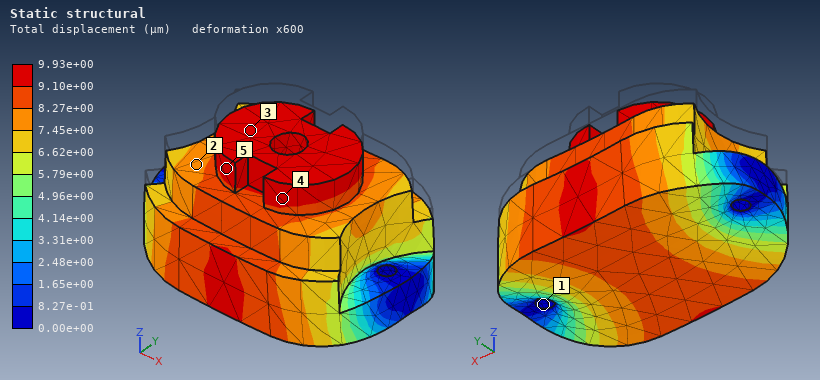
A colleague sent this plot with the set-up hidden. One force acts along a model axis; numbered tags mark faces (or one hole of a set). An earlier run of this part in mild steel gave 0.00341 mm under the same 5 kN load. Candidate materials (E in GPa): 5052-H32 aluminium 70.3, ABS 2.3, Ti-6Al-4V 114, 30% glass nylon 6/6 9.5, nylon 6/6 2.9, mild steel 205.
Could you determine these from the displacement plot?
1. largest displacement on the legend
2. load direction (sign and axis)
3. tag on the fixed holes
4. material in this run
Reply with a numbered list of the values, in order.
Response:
1. 9.93e+00 µm
2. -Z
3. 1
4. 5052-H32 aluminium
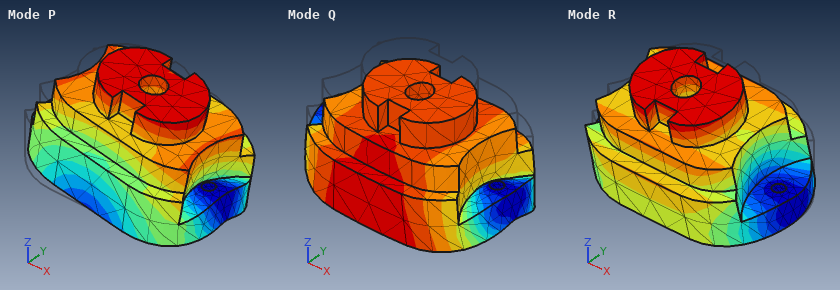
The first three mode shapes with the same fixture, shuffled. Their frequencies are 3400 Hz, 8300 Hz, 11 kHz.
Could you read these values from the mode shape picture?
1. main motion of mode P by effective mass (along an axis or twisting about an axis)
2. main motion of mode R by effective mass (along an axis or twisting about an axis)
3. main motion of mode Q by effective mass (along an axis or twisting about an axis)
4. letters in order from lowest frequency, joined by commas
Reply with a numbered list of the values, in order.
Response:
1. along X
2. along Y
3. along Z
4. R, Q, P
